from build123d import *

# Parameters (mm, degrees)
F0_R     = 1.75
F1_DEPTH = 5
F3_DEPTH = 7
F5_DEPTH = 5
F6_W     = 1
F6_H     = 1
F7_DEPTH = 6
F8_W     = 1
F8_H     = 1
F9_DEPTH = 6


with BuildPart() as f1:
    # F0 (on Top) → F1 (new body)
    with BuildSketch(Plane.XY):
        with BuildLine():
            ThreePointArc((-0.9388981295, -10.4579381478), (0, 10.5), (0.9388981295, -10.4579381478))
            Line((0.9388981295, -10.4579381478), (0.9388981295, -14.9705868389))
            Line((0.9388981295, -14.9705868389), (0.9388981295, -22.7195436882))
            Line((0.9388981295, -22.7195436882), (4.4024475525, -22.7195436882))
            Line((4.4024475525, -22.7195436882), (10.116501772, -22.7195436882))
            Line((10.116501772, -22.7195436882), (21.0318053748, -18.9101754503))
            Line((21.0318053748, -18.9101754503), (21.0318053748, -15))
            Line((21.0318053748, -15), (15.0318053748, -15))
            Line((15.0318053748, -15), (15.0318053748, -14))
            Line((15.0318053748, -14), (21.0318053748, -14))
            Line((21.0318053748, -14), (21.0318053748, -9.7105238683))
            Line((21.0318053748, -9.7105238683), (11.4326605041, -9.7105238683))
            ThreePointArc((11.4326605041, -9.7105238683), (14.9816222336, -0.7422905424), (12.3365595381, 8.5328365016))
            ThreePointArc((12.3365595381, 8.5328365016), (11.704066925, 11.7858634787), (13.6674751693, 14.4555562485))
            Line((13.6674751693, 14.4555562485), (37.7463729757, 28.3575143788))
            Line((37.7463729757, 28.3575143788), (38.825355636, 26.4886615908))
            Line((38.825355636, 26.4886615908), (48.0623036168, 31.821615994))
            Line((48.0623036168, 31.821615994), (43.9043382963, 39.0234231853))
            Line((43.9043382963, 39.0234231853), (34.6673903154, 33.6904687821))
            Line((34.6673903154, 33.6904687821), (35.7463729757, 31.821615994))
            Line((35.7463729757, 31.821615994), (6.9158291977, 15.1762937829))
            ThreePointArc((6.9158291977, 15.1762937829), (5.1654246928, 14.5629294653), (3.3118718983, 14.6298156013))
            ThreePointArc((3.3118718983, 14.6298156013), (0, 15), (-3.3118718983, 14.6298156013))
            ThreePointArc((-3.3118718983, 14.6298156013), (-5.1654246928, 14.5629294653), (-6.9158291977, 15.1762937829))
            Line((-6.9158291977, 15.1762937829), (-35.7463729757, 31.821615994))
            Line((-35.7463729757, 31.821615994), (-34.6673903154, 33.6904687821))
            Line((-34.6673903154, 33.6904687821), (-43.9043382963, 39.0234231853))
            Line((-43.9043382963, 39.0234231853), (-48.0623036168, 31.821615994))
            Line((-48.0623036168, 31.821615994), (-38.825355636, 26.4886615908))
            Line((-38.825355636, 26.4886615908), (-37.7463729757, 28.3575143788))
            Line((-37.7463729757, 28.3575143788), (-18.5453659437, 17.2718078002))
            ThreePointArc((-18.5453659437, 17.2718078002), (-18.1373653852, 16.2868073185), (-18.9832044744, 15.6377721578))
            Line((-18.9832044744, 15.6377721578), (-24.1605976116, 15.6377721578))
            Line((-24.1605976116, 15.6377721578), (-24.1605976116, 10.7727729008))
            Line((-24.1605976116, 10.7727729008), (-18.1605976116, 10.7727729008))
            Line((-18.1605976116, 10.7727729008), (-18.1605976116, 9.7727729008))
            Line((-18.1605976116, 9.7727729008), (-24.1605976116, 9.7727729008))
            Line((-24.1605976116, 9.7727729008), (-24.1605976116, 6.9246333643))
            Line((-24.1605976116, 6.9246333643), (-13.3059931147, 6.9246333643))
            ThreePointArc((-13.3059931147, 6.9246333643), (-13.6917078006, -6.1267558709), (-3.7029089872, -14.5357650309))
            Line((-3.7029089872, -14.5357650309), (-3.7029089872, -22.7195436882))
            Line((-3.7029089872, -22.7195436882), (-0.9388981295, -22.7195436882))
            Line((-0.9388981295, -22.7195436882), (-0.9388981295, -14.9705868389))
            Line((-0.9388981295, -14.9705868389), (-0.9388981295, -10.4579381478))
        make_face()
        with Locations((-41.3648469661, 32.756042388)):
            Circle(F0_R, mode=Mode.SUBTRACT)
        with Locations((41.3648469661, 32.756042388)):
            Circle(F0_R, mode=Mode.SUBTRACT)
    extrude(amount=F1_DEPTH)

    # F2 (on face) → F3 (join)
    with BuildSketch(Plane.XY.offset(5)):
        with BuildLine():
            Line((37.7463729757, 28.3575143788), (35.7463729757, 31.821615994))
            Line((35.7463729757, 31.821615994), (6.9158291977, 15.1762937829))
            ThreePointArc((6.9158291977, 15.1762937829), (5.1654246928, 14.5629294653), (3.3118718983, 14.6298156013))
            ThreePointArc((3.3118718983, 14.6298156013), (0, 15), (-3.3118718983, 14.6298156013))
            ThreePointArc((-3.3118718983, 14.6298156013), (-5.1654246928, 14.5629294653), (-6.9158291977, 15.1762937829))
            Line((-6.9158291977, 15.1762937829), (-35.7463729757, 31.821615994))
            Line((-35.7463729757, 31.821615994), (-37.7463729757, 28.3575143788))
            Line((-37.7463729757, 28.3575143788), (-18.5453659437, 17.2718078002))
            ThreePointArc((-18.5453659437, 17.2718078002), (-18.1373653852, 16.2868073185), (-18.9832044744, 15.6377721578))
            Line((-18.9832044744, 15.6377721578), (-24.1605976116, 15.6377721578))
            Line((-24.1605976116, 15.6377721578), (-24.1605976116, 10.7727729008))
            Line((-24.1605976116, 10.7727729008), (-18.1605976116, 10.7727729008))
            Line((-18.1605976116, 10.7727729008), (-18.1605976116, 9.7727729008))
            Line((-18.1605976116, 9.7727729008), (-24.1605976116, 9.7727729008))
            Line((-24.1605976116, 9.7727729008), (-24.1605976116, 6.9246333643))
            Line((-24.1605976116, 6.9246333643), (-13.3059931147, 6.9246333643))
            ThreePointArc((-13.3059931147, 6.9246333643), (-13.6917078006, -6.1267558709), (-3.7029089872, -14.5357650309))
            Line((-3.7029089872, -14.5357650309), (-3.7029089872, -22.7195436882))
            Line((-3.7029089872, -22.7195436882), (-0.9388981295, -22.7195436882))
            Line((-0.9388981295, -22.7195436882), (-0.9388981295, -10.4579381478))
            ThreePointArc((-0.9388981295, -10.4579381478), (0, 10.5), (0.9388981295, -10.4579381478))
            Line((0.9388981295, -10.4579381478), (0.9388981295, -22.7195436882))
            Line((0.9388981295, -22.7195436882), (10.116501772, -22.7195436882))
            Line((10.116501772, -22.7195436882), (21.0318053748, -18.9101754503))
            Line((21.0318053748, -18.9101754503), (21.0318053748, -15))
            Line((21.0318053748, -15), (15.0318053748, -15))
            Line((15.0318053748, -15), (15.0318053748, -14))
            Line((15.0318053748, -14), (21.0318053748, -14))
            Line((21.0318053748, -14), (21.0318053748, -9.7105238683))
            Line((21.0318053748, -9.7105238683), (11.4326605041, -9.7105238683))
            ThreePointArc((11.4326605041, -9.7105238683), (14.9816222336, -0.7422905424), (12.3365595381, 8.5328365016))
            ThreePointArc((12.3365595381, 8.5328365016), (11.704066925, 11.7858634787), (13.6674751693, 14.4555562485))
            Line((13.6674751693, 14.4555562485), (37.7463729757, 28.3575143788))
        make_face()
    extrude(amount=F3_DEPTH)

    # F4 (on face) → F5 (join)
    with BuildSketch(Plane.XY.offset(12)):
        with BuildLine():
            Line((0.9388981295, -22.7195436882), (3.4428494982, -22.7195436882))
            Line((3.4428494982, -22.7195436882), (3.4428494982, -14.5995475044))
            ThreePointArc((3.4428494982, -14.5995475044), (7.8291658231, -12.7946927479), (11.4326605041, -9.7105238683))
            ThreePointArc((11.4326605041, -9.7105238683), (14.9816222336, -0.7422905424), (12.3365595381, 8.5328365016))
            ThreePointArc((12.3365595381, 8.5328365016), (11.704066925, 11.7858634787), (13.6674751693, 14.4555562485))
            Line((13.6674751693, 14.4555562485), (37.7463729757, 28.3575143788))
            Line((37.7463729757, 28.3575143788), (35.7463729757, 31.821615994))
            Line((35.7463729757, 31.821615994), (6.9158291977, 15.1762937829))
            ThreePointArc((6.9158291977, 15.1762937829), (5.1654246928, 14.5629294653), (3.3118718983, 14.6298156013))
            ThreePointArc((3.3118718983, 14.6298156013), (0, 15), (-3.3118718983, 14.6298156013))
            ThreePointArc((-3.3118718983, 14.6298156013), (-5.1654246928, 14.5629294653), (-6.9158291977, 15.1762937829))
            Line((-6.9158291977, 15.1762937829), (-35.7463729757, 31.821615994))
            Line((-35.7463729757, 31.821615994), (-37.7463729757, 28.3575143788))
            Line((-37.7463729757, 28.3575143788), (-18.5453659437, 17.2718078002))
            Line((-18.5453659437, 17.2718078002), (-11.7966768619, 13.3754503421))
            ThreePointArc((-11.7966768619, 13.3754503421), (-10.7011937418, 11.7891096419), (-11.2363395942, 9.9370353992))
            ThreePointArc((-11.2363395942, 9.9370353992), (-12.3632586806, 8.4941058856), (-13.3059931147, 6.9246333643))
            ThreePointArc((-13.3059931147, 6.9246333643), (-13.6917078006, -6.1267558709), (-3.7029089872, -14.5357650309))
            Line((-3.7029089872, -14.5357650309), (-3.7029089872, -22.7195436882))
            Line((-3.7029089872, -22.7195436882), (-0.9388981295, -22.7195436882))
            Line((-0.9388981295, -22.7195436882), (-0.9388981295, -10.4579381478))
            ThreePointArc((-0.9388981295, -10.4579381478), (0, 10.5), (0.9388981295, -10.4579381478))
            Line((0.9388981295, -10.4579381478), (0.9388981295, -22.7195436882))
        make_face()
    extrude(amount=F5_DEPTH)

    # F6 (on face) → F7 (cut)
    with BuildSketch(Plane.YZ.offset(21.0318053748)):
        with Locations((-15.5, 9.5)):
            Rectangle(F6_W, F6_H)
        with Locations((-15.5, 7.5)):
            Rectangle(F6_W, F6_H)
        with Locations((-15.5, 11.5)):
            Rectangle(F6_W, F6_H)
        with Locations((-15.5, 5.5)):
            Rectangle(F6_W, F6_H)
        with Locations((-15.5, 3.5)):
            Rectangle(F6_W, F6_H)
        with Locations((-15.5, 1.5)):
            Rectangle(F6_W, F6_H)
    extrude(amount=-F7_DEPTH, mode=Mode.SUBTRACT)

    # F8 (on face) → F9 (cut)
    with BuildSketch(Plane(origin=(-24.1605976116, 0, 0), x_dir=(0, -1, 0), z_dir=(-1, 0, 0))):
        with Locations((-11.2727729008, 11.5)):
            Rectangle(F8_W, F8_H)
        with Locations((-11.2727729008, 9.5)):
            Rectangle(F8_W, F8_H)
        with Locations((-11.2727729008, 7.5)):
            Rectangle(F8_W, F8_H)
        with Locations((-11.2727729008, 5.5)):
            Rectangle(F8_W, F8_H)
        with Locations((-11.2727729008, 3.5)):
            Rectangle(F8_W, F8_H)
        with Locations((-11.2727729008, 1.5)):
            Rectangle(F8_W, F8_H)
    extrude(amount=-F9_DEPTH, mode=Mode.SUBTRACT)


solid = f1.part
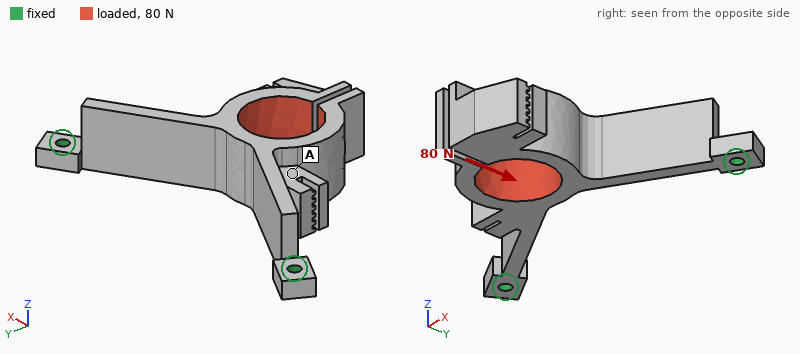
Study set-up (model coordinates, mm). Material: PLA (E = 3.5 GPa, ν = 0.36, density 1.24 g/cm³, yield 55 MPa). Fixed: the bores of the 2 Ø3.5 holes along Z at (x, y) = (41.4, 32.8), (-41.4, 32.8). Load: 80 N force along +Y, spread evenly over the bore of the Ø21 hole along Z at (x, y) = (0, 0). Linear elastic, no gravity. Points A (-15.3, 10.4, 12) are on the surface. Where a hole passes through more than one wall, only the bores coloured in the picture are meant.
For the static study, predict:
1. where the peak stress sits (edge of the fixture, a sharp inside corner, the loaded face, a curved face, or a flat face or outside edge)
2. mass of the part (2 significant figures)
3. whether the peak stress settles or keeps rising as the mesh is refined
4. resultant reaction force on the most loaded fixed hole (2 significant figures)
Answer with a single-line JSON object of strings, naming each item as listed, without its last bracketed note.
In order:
{"where the peak stress sits": "a sharp inside corner", "mass of the part": "19 g", "whether the peak stress settles or keeps rising as the mesh is refined": "keeps rising", "resultant reaction force on the most loaded fixed hole": "72 N"}
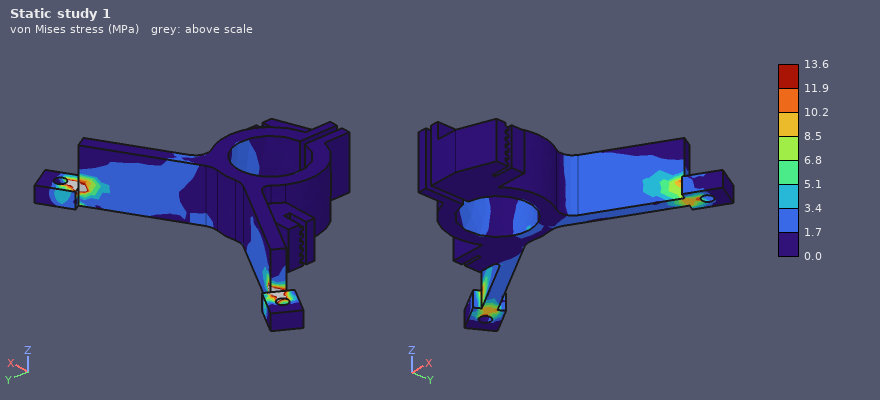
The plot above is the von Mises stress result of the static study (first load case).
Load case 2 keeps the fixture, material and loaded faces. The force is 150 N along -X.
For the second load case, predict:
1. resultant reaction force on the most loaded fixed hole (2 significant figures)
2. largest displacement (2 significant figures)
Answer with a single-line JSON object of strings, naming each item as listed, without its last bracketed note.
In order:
{"resultant reaction force on the most loaded fixed hole": "100 N", "largest displacement": "0.67 mm"}
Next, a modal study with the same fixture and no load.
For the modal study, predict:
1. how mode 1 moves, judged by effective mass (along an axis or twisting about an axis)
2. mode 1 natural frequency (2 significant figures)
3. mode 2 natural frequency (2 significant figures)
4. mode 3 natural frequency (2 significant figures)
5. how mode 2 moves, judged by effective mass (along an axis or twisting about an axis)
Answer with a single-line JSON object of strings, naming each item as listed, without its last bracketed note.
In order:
{"how mode 1 moves, judged by effective mass": "along Z", "mode 1 natural frequency": "200 Hz", "mode 2 natural frequency": "510 Hz", "mode 3 natural frequency": "940 Hz", "how mode 2 moves, judged by effective mass": "along X"}
